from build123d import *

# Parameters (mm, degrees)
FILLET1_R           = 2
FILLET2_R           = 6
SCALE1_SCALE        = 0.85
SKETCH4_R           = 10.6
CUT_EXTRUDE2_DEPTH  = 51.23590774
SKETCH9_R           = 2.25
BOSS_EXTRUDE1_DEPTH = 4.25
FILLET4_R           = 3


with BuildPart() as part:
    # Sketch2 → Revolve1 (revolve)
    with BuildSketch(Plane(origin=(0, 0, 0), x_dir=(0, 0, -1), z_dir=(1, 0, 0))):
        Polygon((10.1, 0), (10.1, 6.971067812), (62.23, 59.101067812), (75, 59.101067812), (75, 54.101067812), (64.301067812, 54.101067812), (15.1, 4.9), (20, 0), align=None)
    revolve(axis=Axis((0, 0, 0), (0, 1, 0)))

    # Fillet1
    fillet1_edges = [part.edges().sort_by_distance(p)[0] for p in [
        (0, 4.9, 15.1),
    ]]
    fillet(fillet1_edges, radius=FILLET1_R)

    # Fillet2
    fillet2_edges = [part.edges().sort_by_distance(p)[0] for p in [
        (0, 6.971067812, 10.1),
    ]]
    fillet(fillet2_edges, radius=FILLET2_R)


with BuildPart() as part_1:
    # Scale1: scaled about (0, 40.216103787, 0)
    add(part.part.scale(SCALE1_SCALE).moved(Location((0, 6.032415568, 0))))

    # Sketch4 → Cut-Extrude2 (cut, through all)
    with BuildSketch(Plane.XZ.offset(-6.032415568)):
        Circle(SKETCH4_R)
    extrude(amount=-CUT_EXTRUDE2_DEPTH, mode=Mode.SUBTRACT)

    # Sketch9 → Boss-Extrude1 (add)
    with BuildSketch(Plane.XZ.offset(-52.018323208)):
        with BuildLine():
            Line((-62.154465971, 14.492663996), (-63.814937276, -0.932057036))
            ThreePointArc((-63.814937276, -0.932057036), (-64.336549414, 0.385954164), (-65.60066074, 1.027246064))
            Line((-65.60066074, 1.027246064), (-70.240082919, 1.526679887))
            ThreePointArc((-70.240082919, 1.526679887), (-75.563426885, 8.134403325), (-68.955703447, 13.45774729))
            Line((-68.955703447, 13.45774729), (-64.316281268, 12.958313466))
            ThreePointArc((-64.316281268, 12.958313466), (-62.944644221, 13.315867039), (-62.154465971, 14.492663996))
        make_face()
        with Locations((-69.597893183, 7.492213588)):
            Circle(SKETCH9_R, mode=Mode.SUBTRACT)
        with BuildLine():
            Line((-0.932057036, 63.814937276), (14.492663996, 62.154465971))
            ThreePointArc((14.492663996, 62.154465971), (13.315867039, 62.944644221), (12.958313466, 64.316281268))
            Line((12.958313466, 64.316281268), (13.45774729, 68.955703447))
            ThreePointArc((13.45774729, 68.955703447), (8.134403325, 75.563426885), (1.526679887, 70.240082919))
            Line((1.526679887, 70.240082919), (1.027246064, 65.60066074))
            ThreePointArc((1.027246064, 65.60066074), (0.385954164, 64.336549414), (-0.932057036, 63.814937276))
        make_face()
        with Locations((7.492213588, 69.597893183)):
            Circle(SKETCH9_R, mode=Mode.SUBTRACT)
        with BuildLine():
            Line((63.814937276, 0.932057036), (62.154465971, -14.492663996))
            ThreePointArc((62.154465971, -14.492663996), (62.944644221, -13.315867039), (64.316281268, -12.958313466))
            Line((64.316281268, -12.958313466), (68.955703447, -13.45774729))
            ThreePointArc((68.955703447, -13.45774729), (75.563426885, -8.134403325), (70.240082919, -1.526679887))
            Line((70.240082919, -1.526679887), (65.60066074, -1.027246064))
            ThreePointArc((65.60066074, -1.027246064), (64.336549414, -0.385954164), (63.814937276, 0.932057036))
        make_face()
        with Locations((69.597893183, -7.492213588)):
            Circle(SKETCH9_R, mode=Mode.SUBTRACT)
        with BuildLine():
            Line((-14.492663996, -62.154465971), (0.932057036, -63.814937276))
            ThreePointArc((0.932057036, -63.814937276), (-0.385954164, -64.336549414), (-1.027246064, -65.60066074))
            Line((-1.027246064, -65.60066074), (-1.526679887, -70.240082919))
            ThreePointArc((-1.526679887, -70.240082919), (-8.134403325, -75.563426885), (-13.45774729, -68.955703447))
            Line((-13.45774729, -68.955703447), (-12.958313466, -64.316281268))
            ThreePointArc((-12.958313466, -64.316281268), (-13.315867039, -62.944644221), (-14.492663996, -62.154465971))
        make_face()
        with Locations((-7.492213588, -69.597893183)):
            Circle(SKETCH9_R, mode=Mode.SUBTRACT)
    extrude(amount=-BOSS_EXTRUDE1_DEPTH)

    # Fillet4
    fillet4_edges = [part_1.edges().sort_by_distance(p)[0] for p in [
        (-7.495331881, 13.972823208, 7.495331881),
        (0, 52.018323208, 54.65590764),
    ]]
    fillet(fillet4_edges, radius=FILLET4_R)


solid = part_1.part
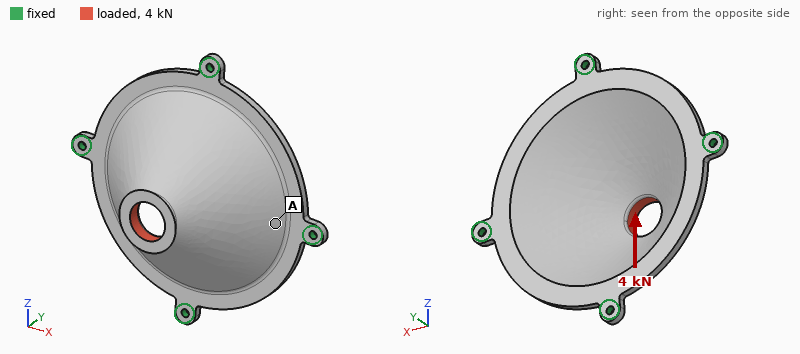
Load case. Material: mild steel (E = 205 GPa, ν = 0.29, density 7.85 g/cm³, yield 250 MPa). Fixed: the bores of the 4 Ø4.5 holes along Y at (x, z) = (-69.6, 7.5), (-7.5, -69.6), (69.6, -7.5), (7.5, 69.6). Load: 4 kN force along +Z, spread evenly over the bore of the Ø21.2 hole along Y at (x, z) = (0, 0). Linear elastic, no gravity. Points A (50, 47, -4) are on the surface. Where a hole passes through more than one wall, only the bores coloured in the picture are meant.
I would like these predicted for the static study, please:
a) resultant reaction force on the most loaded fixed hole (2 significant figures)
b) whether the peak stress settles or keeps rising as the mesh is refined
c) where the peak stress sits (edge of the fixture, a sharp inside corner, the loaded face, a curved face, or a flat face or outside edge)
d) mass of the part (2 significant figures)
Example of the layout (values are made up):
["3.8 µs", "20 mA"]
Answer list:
["2.5 kN", "keeps rising", "edge of the fixture", "560 g"]
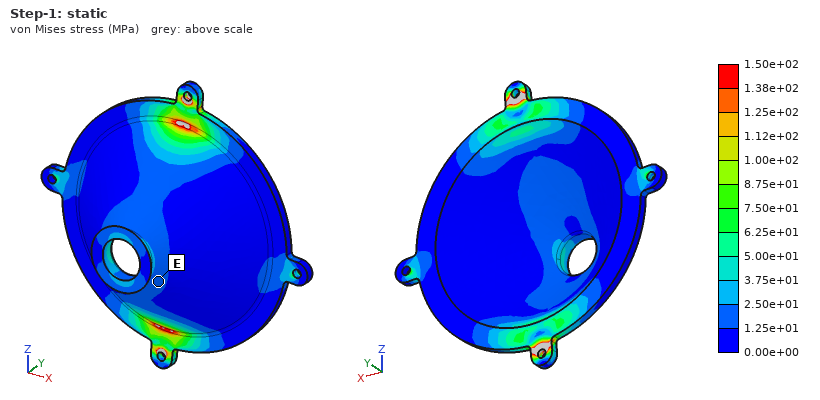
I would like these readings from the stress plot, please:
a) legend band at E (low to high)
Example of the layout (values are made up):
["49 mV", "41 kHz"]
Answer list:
["1.25e+01 to 2.50e+01 MPa"]
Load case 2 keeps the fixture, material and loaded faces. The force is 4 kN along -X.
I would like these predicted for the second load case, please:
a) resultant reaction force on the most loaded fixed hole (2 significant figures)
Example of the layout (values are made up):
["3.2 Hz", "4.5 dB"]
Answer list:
["2.5 kN"]
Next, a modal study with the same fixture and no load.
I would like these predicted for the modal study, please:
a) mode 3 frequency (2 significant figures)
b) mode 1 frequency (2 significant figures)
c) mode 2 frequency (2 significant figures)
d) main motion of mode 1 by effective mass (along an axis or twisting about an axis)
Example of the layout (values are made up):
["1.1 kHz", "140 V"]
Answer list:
["3000 Hz", "2600 Hz", "3000 Hz", "along Y"]
